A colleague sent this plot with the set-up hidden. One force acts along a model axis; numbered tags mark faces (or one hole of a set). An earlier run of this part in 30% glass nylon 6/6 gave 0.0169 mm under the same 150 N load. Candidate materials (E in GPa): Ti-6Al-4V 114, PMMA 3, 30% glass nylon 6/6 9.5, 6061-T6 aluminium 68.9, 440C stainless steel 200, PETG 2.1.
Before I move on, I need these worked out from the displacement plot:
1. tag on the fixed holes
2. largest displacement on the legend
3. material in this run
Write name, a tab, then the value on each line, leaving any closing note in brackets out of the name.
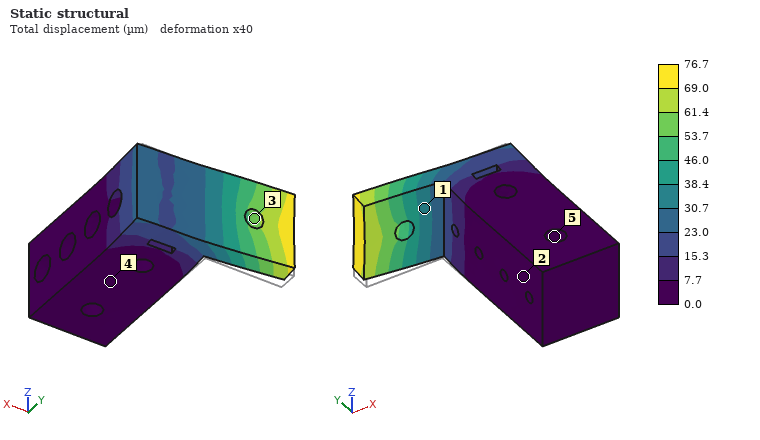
tag on the fixed holes	5
largest displacement on the legend	76.7 µm
material in this run	PETG
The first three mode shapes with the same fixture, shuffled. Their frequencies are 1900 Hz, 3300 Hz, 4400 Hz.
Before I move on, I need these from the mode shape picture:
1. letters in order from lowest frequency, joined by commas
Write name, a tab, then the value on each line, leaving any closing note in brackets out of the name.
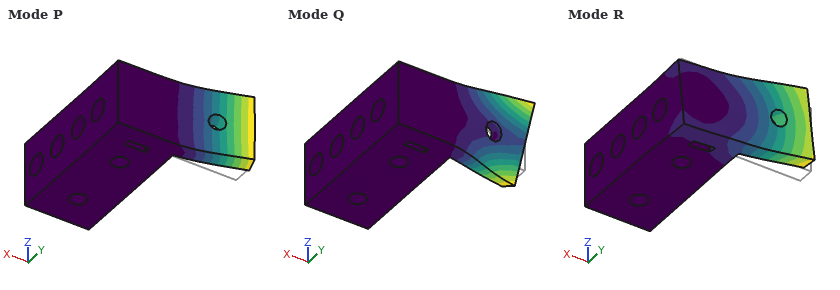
letters in order from lowest frequency, joined by commas	P, R, Q
